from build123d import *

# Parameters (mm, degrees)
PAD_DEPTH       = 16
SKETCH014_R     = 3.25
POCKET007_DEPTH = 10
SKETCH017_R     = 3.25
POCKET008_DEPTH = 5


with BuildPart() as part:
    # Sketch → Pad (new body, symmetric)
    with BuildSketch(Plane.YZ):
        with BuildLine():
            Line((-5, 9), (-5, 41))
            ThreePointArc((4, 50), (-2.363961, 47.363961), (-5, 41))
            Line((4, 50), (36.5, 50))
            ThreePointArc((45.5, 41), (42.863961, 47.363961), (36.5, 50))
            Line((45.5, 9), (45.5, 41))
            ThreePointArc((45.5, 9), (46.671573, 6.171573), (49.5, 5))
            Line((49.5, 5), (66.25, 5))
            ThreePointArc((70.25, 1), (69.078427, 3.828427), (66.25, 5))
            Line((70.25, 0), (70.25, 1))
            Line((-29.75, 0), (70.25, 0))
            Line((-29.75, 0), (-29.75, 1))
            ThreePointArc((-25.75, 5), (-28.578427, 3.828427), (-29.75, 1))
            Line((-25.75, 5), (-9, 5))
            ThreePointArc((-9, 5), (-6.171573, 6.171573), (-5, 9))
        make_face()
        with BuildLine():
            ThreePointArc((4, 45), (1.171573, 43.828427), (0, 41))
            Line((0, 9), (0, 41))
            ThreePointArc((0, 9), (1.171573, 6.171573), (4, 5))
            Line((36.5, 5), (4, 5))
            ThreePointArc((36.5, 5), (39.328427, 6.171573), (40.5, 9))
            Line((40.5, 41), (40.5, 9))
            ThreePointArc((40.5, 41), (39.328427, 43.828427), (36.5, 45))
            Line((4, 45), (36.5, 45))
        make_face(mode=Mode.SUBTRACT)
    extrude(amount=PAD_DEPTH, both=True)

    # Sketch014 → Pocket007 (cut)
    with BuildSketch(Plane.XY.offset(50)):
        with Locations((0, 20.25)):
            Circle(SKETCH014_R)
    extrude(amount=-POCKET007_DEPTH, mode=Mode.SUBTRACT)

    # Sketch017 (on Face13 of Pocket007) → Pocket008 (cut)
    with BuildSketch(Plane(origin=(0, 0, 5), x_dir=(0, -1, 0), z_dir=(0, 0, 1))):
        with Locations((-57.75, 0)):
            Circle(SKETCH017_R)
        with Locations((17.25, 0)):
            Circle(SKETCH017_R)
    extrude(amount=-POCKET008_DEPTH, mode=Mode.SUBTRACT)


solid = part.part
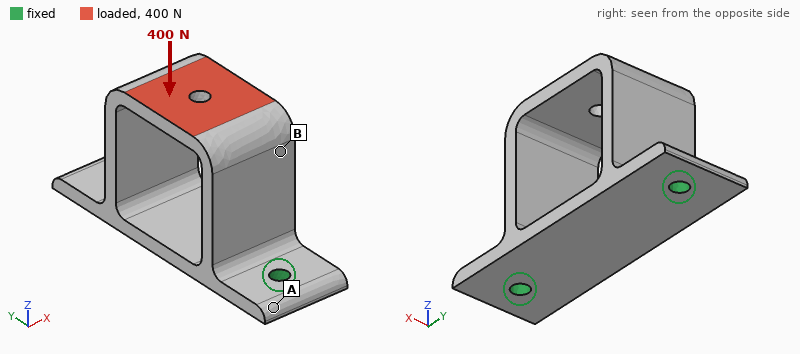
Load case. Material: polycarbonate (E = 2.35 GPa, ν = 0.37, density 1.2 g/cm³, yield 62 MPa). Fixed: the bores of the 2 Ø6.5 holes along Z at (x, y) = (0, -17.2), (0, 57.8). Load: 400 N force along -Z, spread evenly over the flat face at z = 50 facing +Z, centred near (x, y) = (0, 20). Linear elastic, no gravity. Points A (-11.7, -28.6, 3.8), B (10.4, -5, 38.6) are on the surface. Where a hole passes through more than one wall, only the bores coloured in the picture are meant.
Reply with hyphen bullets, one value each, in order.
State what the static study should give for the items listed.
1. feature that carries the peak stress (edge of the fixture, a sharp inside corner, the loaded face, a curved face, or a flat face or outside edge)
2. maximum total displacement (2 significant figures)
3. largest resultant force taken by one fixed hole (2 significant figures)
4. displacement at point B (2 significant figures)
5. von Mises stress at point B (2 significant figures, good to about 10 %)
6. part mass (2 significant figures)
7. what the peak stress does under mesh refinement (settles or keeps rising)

- edge of the fixture
- 0.44 mm
- 210 N
- 0.14 mm
- 5.4 MPa
- 43 g
- keeps rising
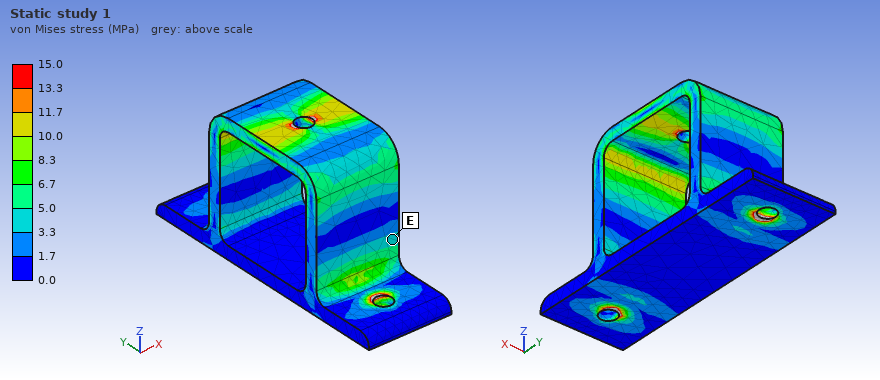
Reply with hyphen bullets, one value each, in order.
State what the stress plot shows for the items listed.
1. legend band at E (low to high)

- 3.3 to 5.0 MPa
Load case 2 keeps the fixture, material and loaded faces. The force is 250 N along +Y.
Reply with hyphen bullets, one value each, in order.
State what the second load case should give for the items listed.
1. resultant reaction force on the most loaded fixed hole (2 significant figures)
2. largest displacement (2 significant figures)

- 210 N
- 1.3 mm
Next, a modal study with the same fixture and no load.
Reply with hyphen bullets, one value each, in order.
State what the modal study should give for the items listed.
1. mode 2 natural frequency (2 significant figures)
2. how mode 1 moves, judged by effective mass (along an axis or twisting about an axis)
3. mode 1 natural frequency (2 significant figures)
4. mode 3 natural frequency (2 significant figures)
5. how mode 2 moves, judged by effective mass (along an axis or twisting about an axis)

- 600 Hz
- along X
- 450 Hz
- 970 Hz
- along Y
